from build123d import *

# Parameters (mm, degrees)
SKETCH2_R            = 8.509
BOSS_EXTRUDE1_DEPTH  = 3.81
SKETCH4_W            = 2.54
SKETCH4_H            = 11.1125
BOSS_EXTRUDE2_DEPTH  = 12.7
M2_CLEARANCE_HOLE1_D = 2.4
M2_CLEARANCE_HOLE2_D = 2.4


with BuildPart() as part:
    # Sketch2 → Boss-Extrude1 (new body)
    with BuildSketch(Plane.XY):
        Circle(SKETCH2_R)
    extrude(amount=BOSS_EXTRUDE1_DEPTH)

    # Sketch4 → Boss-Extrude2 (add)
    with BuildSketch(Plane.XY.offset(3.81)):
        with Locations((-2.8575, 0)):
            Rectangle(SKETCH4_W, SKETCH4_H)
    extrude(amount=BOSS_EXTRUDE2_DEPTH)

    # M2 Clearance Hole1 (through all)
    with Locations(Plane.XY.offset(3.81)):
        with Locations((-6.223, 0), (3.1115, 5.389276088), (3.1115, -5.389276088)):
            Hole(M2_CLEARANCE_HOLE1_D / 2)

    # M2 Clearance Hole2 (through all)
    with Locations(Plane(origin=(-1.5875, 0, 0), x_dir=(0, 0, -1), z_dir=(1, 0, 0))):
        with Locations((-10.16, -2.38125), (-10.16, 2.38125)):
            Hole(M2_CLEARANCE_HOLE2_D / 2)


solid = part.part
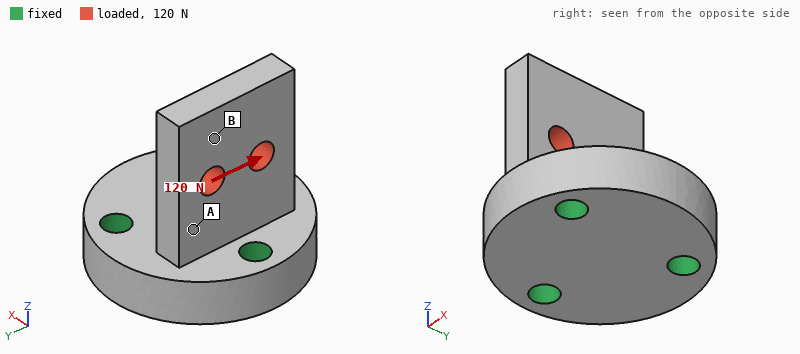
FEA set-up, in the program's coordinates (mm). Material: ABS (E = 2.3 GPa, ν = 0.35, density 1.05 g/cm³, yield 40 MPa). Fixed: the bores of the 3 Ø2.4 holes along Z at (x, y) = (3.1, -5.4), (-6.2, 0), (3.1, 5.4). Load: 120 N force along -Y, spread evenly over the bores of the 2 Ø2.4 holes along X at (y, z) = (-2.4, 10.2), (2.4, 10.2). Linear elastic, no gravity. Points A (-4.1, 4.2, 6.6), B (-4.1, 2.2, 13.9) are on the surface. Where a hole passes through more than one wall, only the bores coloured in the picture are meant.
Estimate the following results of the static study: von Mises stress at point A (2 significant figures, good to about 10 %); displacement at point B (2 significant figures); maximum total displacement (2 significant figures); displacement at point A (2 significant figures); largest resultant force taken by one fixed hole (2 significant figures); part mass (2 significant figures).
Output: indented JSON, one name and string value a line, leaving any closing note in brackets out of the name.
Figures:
{
  "von Mises stress at point A": "6.6 MPa",
  "displacement at point B": "0.16 mm",
  "maximum total displacement": "0.19 mm",
  "displacement at point A": "0.063 mm",
  "largest resultant force taken by one fixed hole": "65 N",
  "part mass": "1.2 g"
}
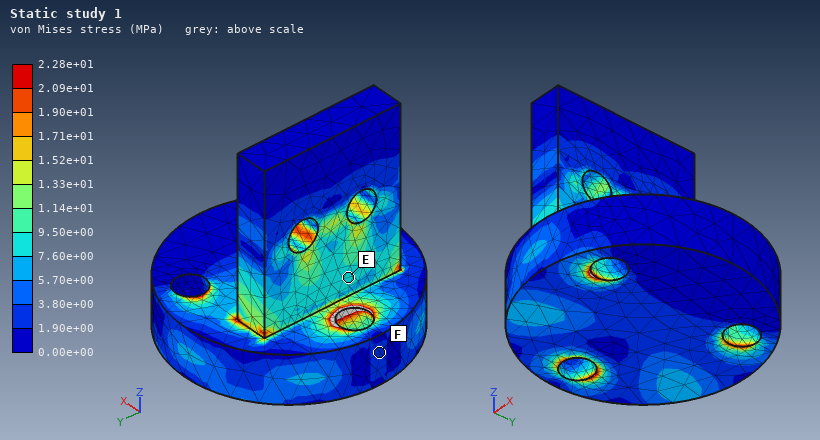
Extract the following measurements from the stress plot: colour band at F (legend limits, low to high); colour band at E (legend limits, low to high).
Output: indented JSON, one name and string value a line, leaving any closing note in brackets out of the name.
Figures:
{
  "colour band at F": "1.90e+00 to 3.80e+00 MPa",
  "colour band at E": "7.60e+00 to 9.50e+00 MPa"
}
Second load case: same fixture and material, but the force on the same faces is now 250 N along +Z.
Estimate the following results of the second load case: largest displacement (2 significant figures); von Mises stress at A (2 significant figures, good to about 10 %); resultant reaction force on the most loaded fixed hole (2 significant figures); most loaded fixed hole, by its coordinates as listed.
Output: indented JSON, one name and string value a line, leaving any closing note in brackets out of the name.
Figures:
{
  "largest displacement": "58 µm",
  "von Mises stress at A": "7.9 MPa",
  "resultant reaction force on the most loaded fixed hole": "150 N",
  "most loaded fixed hole, by its coordinates as listed": "(-6.2, 0)"
}
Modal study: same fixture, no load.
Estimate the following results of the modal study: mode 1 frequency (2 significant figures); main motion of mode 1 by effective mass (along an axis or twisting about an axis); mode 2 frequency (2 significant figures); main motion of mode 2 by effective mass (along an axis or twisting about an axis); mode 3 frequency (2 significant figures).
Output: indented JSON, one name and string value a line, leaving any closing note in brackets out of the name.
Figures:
{
  "mode 1 frequency": "3200 Hz",
  "main motion of mode 1 by effective mass": "along X",
  "mode 2 frequency": "7400 Hz",
  "main motion of mode 2 by effective mass": "along Y",
  "mode 3 frequency": "7900 Hz"
}
